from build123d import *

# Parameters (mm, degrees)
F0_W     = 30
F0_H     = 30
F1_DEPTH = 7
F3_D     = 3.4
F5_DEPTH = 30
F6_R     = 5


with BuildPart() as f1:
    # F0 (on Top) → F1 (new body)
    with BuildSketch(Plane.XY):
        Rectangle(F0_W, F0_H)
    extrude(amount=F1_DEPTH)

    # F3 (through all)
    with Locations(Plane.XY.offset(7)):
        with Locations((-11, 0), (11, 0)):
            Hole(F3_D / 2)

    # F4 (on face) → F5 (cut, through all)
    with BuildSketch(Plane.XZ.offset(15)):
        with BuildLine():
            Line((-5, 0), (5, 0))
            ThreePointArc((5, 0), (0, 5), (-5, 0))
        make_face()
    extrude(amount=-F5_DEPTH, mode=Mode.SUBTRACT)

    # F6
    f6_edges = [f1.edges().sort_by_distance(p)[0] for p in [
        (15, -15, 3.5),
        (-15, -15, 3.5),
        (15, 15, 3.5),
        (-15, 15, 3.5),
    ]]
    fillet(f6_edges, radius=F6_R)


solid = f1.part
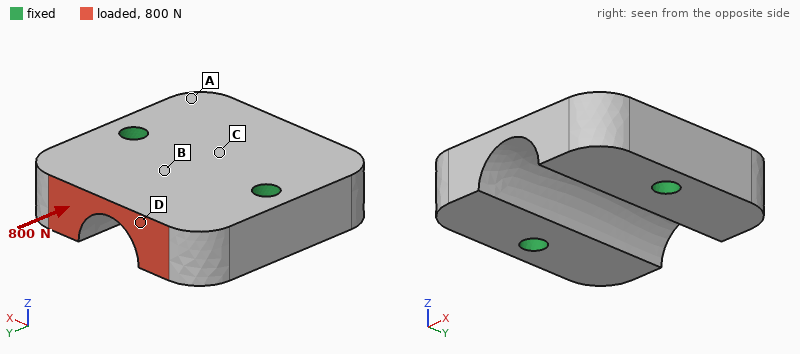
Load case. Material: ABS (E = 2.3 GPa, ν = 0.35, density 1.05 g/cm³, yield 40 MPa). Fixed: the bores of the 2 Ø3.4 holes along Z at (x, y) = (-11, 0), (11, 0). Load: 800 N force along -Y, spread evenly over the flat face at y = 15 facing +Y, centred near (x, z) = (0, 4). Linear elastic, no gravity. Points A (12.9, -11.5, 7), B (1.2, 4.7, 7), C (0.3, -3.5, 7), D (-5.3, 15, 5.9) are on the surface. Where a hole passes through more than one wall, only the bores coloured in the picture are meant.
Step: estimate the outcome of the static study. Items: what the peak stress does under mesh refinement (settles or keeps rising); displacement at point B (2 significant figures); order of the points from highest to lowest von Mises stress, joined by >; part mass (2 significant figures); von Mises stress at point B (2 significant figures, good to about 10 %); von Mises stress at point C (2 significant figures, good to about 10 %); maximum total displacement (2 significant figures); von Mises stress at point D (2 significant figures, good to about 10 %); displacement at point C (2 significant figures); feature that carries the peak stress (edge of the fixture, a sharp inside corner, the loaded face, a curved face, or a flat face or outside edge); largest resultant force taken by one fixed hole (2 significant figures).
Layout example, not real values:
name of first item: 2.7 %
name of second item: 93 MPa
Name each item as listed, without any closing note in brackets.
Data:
what the peak stress does under mesh refinement: keeps rising
displacement at point B: 48 µm
order of the points from highest to lowest von Mises stress, joined by >: D > B > C > A
part mass: 5.1 g
von Mises stress at point B: 5.6 MPa
von Mises stress at point C: 3.0 MPa
maximum total displacement: 96 µm
von Mises stress at point D: 7.9 MPa
displacement at point C: 27 µm
feature that carries the peak stress: edge of the fixture
largest resultant force taken by one fixed hole: 410 N
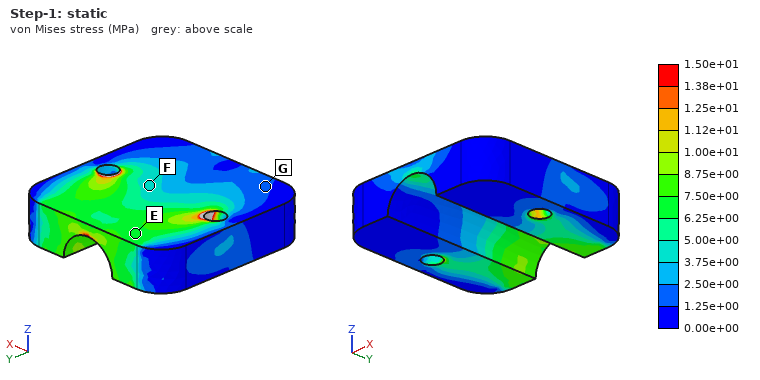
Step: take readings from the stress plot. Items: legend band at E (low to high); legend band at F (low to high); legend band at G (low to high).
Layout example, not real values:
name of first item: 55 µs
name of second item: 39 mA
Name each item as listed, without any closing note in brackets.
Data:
legend band at E: 6.25e+00 to 7.50e+00 MPa
legend band at F: 3.75e+00 to 5.00e+00 MPa
legend band at G: 1.25e+00 to 2.50e+00 MPa
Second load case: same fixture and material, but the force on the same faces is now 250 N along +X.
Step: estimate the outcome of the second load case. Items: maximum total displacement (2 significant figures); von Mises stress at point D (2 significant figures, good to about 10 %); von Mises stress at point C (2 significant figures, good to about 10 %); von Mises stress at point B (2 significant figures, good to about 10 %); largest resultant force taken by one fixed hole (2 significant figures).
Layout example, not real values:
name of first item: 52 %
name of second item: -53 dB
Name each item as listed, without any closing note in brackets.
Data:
maximum total displacement: 75 µm
von Mises stress at point D: 5.7 MPa
von Mises stress at point C: 1.6 MPa
von Mises stress at point B: 5.1 MPa
largest resultant force taken by one fixed hole: 190 N
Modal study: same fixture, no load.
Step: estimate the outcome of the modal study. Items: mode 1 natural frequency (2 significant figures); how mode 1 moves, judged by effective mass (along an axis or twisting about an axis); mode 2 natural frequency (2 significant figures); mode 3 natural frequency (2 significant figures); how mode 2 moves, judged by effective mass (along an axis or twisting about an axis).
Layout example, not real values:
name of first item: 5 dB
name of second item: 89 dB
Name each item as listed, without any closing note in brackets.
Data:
mode 1 natural frequency: 5800 Hz
how mode 1 moves, judged by effective mass: twisting about X
mode 2 natural frequency: 7100 Hz
mode 3 natural frequency: 7600 Hz
how mode 2 moves, judged by effective mass: along Z
